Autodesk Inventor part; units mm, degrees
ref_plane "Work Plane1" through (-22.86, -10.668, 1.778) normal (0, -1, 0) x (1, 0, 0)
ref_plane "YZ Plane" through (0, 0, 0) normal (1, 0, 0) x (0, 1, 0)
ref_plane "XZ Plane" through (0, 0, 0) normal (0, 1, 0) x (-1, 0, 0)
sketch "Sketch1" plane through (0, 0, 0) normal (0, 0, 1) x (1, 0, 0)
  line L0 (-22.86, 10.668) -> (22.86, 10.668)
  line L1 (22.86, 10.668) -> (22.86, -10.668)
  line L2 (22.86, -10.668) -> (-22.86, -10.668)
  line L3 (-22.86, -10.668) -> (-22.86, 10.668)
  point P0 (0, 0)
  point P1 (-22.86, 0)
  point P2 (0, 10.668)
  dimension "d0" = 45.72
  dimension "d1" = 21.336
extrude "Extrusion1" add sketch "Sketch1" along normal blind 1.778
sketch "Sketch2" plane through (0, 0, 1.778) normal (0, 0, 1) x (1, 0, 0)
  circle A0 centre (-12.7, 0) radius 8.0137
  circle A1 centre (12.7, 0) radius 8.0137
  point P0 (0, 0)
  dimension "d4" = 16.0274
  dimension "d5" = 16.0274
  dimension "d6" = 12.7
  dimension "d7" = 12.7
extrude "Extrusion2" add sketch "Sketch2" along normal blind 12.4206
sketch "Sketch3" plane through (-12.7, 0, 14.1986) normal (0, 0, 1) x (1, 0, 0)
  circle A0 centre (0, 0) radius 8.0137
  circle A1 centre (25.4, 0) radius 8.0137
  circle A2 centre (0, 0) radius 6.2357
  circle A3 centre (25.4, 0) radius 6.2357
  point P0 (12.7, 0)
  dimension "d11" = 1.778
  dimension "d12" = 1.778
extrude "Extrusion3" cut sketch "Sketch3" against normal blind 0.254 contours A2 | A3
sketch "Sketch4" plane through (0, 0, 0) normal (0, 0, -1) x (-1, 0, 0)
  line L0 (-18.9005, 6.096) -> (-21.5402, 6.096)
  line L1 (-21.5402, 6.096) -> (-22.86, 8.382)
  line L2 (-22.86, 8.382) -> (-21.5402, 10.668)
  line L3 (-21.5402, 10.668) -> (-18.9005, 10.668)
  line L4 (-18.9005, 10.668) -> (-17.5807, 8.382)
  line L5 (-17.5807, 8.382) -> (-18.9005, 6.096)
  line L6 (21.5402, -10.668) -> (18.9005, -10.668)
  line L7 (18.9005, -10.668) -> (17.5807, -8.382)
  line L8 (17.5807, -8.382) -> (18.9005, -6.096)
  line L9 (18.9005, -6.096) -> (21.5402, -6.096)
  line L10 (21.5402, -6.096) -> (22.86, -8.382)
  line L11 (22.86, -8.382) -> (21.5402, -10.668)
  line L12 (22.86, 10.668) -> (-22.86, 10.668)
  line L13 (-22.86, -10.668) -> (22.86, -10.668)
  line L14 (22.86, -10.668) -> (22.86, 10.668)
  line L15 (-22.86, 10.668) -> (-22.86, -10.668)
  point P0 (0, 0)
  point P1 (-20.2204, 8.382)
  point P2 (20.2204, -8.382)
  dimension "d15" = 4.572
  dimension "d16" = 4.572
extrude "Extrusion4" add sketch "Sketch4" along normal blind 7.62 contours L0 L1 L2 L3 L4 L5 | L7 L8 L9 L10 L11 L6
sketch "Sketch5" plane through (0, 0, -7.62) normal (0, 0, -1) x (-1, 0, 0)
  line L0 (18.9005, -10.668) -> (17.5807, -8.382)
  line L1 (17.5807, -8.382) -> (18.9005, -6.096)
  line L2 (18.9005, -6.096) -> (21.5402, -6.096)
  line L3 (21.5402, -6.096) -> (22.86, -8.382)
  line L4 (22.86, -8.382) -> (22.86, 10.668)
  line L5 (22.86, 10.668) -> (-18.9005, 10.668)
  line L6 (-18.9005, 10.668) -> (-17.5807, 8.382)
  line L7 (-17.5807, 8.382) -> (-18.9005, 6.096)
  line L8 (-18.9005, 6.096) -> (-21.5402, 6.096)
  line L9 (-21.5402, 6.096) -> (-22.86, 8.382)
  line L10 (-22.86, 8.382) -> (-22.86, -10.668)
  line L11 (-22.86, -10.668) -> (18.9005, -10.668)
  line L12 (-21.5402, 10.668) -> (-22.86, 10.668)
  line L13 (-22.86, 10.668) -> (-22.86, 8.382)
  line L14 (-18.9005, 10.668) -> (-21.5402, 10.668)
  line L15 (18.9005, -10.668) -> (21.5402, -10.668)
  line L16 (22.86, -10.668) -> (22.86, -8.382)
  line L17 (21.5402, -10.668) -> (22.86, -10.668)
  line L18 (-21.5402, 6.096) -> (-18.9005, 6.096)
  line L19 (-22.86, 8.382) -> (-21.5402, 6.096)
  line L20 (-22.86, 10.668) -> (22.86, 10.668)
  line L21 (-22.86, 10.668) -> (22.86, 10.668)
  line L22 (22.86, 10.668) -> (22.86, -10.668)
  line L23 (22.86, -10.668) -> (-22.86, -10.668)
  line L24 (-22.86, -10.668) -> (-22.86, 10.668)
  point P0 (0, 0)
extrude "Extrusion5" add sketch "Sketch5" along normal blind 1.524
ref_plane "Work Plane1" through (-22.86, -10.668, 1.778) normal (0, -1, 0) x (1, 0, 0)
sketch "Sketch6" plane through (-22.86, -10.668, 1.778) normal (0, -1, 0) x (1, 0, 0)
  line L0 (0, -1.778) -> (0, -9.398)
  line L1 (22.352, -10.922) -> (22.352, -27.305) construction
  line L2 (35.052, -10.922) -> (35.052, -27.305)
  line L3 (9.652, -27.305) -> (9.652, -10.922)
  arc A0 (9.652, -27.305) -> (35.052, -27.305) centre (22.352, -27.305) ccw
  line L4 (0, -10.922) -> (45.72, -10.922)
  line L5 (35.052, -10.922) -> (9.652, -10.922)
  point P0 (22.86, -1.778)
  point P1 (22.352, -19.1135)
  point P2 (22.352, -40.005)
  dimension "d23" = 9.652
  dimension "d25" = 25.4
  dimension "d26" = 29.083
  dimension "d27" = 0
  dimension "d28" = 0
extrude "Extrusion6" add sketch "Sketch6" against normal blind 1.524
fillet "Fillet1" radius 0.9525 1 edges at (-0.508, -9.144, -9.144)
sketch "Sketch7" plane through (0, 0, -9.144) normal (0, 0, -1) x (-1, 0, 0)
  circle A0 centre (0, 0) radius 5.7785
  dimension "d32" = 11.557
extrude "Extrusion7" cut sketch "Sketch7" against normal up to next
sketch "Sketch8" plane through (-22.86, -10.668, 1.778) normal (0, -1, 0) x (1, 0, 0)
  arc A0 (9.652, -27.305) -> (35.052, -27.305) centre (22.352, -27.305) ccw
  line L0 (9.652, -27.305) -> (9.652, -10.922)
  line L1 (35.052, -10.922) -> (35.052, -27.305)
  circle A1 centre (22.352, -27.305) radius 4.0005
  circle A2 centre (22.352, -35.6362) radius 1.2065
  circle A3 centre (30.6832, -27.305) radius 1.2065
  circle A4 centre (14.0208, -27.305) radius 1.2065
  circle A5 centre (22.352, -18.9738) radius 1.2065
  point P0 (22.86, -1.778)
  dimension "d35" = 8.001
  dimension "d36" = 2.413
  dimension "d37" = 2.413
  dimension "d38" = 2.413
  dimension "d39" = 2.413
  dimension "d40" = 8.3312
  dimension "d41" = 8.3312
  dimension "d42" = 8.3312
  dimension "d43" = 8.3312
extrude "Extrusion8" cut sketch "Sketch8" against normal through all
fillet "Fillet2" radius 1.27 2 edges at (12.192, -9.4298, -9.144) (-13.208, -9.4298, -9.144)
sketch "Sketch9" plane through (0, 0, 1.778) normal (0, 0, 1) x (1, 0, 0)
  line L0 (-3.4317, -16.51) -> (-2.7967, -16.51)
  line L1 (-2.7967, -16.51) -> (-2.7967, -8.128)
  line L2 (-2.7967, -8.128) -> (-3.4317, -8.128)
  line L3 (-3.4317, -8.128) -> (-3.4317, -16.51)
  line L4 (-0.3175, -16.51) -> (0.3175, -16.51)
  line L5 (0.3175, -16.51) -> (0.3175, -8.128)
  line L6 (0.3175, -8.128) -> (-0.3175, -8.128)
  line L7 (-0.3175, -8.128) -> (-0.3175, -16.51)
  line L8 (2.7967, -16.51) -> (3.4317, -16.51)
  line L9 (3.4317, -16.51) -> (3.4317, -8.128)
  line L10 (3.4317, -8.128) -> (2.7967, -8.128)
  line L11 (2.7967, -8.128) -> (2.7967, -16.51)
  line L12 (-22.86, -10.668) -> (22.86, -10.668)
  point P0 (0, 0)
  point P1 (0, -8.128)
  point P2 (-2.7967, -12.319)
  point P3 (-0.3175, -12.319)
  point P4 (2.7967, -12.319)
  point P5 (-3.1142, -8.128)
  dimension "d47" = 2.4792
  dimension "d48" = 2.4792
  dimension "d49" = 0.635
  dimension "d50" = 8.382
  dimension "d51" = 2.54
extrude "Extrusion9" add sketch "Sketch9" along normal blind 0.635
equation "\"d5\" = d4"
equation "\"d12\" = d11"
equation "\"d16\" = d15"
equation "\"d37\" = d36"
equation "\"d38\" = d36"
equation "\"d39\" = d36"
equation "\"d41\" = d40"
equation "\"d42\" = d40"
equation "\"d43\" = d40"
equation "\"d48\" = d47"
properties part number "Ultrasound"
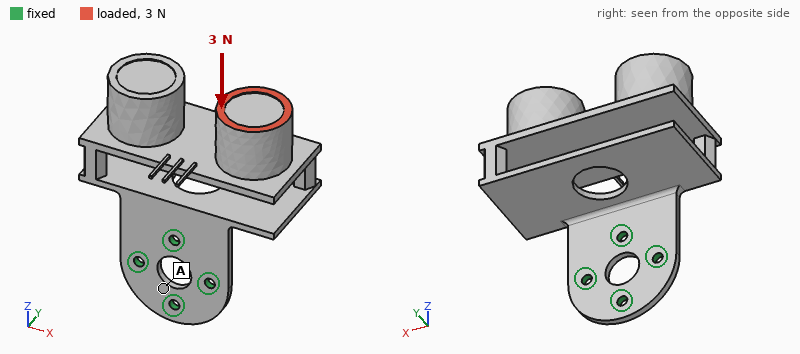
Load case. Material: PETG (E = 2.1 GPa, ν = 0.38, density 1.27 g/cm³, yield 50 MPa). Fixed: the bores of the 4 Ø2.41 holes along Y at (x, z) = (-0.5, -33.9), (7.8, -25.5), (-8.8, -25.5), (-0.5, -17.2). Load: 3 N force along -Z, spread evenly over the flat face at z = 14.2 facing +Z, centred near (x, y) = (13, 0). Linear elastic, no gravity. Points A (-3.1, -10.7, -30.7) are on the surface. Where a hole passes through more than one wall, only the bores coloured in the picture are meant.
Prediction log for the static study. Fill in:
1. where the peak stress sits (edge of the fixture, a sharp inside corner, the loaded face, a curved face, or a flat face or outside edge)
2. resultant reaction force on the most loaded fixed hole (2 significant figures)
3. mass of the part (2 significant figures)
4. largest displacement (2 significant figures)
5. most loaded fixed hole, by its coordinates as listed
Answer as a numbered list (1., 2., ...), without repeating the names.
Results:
1. a curved face
2. 3.1 N
3. 12 g
4. 0.76 mm
5. (7.8, -25.5)
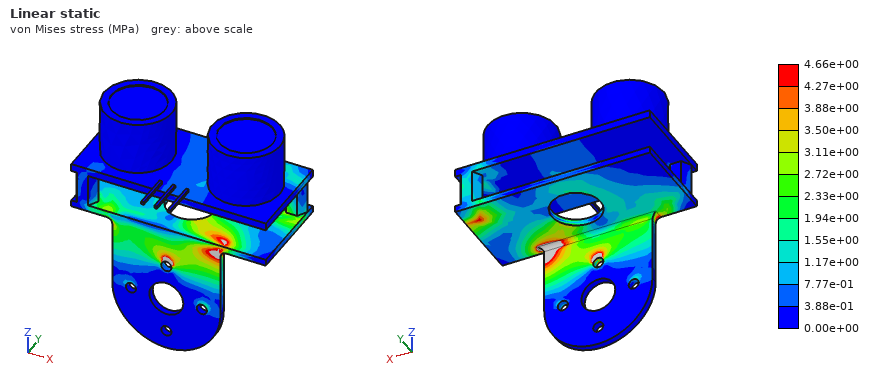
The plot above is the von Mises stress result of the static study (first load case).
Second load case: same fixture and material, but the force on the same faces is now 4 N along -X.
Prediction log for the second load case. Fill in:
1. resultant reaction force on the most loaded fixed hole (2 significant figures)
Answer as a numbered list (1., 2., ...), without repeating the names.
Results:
1. 6.1 N
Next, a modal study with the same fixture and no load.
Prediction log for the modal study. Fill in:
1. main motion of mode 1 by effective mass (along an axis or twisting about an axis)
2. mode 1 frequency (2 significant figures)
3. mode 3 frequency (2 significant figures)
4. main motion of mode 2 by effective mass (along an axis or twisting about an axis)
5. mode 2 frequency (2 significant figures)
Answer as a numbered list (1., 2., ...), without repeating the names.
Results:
1. along Y
2. 80 Hz
3. 180 Hz
4. along X
5. 170 Hz
